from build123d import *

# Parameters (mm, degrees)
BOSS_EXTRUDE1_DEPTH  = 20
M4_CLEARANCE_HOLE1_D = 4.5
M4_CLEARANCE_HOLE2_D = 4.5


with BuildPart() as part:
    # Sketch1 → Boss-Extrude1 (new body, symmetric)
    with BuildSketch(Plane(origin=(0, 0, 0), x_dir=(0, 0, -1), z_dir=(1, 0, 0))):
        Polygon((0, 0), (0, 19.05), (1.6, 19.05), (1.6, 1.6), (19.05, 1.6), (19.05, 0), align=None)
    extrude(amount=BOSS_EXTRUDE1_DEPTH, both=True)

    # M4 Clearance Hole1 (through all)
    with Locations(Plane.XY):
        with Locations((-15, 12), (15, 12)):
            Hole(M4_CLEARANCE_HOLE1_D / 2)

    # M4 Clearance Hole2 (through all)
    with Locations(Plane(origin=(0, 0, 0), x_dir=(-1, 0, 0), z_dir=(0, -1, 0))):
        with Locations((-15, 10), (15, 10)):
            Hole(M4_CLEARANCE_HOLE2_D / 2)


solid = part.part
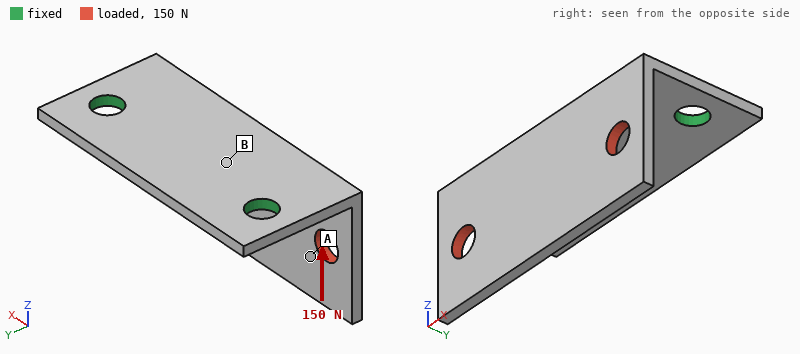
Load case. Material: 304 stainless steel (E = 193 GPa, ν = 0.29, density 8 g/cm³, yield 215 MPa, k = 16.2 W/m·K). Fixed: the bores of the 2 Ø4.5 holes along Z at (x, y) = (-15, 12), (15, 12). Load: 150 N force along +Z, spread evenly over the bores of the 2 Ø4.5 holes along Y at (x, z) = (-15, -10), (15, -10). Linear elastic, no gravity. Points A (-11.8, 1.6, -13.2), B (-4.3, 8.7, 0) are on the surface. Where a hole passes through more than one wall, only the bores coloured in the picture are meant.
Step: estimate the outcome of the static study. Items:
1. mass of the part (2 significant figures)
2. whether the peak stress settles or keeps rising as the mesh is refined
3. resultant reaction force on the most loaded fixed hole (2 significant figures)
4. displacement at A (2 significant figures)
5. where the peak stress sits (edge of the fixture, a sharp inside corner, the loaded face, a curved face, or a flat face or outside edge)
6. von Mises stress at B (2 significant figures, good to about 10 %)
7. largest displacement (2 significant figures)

18 g
keeps rising
75 N
45 µm
edge of the fixture
29 MPa
64 µm
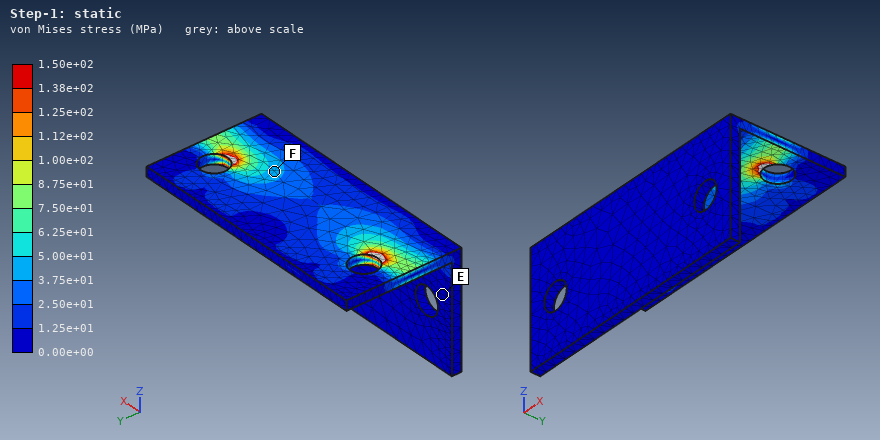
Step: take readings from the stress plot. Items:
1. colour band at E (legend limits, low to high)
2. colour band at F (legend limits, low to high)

0.00e+00 to 1.25e+01 MPa
3.75e+01 to 5.00e+01 MPa
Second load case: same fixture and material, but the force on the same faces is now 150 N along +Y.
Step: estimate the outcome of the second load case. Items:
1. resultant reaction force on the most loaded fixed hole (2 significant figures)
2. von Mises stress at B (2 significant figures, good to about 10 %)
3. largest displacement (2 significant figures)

75 N
45 MPa
0.14 mm
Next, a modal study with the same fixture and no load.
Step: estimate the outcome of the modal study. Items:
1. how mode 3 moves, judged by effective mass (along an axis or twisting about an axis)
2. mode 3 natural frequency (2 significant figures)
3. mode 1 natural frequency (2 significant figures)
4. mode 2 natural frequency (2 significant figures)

along Z
5800 Hz
2000 Hz
3800 Hz
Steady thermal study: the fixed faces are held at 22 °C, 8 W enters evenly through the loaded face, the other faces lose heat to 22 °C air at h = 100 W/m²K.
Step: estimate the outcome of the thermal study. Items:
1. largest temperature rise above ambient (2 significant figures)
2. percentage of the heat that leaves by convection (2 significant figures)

77 K
83 %
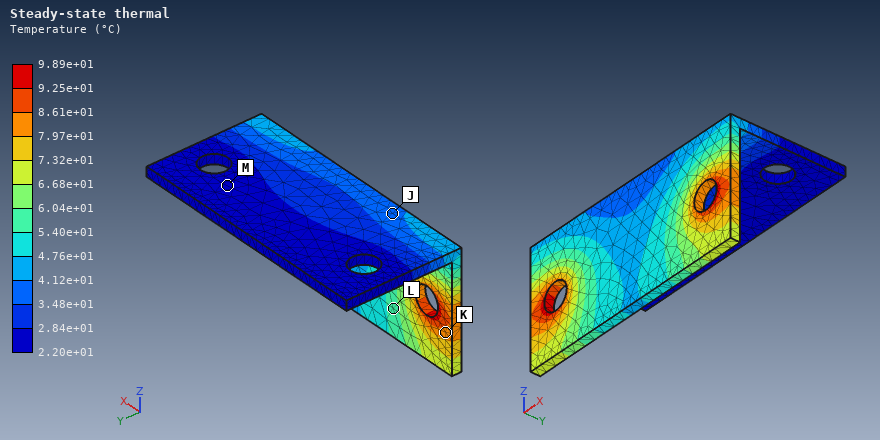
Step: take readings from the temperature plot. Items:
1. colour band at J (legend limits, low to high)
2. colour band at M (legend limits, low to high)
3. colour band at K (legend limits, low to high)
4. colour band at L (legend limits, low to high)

3.48e+01 to 4.12e+01 °C
2.20e+01 to 2.84e+01 °C
7.97e+01 to 8.61e+01 °C
5.40e+01 to 6.04e+01 °C
